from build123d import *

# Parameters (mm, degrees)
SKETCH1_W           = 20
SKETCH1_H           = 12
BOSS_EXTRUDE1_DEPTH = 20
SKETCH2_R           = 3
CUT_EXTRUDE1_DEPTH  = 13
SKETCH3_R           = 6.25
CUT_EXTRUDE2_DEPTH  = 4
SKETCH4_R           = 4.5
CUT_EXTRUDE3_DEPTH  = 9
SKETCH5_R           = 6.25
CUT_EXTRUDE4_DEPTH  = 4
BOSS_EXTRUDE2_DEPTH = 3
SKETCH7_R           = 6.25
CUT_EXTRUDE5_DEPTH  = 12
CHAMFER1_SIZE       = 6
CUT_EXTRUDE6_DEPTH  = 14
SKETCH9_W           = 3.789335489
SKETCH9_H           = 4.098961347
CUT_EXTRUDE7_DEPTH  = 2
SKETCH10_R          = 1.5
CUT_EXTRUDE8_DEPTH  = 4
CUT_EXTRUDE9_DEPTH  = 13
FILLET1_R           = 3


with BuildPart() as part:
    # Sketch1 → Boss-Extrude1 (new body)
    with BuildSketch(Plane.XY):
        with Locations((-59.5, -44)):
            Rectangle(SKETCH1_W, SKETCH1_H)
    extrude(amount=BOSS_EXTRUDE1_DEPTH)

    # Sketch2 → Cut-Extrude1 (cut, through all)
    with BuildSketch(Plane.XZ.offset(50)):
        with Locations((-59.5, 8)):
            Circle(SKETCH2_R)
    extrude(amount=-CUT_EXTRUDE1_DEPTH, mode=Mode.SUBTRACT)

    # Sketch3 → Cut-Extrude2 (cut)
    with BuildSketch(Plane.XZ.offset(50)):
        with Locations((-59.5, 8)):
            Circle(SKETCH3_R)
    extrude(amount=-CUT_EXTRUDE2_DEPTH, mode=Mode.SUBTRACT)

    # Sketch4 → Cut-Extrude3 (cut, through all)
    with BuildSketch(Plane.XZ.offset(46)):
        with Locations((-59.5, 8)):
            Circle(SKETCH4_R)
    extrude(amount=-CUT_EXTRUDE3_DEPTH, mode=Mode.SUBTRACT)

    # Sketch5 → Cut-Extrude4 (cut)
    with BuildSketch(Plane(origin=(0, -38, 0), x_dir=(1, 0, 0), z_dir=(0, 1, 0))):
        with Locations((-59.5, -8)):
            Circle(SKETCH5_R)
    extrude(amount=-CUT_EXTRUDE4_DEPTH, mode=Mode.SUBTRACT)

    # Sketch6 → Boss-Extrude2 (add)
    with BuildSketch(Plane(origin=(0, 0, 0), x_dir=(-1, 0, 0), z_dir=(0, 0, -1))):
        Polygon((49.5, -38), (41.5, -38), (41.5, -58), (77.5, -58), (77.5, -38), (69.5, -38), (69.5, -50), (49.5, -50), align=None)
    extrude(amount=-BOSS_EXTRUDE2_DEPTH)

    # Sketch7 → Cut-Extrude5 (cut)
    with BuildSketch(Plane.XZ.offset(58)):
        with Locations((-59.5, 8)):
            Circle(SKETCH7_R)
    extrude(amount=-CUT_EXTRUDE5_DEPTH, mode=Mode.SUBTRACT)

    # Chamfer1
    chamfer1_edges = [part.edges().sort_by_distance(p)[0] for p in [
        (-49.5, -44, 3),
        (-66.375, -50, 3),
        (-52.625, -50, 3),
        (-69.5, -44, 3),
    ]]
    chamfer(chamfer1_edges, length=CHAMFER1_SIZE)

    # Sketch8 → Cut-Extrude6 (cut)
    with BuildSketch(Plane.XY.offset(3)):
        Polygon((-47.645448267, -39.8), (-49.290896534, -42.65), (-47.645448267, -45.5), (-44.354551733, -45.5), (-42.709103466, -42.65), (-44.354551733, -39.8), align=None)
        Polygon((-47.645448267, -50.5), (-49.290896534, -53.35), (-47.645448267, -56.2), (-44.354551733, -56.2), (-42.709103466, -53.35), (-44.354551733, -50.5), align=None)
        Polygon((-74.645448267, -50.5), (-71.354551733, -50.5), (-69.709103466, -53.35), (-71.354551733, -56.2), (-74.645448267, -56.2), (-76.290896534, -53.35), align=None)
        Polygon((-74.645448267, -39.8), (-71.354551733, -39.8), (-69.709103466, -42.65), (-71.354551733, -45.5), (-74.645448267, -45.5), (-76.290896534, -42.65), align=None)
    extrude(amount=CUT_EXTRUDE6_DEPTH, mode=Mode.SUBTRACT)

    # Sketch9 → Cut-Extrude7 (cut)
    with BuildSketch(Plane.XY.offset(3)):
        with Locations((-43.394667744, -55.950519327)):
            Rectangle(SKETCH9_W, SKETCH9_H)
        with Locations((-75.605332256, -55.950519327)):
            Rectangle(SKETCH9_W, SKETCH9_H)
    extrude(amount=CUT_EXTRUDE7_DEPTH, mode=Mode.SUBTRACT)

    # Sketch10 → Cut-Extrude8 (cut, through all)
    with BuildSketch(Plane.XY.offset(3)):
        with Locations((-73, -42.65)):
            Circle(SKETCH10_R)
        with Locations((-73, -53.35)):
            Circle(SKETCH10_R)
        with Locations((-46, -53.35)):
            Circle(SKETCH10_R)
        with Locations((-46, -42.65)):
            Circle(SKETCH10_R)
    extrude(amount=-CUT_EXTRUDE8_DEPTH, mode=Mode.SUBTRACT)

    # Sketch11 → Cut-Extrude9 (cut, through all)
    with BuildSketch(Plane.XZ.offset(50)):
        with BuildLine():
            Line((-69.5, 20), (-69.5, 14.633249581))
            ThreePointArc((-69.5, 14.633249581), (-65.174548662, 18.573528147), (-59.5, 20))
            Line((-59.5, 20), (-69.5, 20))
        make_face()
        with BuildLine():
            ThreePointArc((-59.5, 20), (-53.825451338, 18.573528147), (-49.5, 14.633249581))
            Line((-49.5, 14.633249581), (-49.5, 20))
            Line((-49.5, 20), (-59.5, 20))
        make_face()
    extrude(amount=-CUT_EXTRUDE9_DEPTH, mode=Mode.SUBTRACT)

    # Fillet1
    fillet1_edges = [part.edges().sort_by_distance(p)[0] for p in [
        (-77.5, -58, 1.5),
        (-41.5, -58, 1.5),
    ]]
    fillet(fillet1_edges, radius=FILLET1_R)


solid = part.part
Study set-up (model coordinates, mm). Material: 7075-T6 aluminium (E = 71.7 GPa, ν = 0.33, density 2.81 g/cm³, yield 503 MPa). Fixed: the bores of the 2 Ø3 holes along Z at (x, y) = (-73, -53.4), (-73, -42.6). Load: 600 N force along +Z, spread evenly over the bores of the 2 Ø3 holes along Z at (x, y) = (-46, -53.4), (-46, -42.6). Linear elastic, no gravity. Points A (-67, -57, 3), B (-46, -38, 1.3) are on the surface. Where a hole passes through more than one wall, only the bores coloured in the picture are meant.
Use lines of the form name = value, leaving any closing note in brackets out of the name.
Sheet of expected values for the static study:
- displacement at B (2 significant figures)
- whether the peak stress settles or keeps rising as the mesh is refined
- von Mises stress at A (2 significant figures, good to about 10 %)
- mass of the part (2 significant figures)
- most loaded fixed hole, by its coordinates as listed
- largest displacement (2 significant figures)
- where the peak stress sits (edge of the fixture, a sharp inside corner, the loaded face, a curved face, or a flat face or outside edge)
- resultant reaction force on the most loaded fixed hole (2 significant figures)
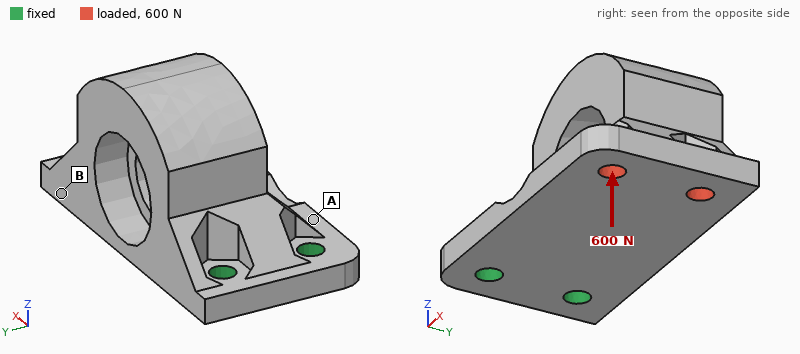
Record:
displacement at B = 0.29 mm
whether the peak stress settles or keeps rising as the mesh is refined = keeps rising
von Mises stress at A = 78 MPa
mass of the part = 14 g
most loaded fixed hole, by its coordinates as listed = (-73, -42.6)
largest displacement = 0.36 mm
where the peak stress sits = edge of the fixture
resultant reaction force on the most loaded fixed hole = 390 N
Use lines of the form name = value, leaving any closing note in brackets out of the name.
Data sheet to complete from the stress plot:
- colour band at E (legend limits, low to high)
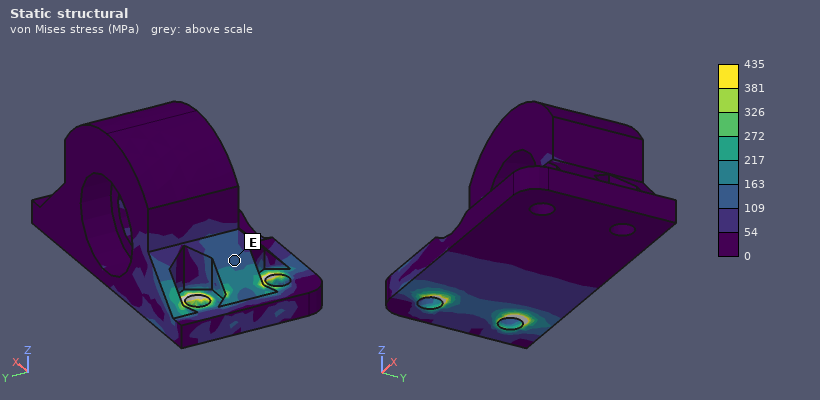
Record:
colour band at E = 109 to 163 MPa
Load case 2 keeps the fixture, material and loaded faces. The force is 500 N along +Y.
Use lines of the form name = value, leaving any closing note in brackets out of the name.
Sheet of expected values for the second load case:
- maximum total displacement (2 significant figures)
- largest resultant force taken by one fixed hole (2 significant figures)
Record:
maximum total displacement = 47 µm
largest resultant force taken by one fixed hole = 1.1 kN
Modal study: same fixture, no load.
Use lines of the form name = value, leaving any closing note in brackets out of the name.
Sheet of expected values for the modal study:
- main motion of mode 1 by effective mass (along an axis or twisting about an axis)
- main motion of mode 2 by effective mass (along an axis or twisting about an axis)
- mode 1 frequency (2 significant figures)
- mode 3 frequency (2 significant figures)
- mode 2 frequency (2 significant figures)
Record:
main motion of mode 1 by effective mass = along Z
main motion of mode 2 by effective mass = along Y
mode 1 frequency = 3000 Hz
mode 3 frequency = 12 kHz
mode 2 frequency = 8200 Hz
